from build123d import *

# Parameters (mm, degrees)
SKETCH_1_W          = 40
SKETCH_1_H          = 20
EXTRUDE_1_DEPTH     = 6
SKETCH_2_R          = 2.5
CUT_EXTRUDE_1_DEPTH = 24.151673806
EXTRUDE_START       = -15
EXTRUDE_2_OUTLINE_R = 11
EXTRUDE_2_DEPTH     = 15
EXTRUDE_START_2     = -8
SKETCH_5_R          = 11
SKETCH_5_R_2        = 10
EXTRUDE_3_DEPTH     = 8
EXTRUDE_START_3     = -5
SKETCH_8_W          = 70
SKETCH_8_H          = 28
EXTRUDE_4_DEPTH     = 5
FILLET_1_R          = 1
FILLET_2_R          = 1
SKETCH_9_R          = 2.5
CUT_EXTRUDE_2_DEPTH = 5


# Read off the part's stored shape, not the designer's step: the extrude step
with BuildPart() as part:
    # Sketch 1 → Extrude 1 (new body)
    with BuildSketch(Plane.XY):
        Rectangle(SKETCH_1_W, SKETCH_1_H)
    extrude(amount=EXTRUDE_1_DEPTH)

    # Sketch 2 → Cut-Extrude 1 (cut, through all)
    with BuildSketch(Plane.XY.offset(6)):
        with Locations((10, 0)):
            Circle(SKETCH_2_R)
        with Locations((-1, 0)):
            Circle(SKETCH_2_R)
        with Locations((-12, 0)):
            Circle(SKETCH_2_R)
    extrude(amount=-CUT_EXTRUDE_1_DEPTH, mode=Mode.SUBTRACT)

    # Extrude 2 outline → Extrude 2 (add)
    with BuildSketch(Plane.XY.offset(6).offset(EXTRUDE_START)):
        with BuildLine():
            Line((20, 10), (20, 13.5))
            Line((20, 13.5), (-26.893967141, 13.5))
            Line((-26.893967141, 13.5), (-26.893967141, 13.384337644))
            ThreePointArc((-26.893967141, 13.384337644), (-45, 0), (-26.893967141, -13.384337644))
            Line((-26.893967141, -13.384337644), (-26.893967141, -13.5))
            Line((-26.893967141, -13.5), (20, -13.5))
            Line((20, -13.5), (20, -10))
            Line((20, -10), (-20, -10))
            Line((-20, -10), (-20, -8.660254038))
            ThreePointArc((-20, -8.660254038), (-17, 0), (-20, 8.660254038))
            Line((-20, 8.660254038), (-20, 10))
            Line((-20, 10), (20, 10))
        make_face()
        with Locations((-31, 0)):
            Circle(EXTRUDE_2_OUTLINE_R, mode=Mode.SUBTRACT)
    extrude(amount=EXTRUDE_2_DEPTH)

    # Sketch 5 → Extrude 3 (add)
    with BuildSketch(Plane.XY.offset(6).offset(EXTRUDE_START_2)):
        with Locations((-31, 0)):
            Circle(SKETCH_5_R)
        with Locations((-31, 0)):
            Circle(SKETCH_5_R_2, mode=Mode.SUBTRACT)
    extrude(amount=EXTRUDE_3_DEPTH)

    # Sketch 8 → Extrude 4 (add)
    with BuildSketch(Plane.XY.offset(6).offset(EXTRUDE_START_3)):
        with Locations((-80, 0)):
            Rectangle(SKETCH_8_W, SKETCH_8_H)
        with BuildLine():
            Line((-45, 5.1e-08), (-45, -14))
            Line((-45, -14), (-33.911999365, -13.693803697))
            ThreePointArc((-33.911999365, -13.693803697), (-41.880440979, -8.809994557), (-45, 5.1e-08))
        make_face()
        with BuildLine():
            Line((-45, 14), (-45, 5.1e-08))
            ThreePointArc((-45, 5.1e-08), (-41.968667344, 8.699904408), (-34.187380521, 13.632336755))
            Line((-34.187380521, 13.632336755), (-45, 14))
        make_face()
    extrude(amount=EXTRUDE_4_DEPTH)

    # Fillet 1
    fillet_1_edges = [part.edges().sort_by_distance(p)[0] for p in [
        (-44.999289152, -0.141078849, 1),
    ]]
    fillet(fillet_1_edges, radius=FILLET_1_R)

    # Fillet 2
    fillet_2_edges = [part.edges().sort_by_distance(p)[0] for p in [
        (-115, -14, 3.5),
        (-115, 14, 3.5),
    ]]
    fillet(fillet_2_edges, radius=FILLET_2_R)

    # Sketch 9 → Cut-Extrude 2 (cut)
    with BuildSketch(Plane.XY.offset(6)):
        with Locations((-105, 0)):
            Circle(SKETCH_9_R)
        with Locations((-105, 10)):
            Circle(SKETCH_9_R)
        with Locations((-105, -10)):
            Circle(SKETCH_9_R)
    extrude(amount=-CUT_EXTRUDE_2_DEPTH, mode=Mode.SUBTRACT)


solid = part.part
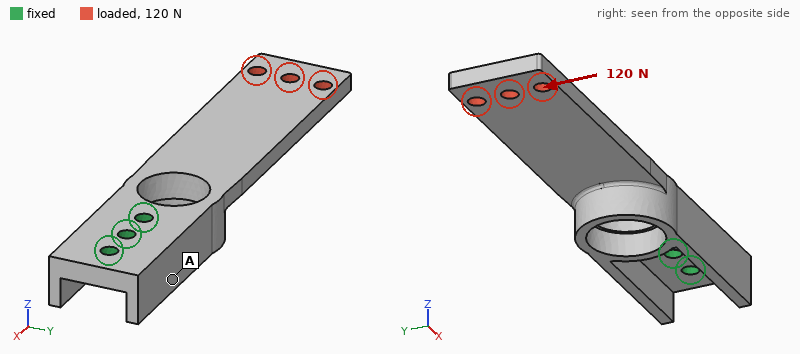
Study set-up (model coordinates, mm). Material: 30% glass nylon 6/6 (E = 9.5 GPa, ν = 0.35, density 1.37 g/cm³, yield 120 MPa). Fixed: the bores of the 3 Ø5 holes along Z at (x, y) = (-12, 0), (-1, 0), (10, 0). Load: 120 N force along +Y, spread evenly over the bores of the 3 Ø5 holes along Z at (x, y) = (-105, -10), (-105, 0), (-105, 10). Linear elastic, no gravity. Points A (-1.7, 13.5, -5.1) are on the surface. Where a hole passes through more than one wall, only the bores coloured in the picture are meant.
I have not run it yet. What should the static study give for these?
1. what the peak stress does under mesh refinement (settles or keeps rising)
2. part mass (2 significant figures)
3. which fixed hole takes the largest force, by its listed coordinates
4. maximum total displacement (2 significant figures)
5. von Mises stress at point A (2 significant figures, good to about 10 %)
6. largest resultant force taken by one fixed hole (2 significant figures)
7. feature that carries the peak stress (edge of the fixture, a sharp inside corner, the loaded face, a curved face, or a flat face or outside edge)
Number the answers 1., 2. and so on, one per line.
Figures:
1. keeps rising
2. 31 g
3. (-12, 0)
4. 0.58 mm
5. 3.2 MPa
6. 550 N
7. edge of the fixture
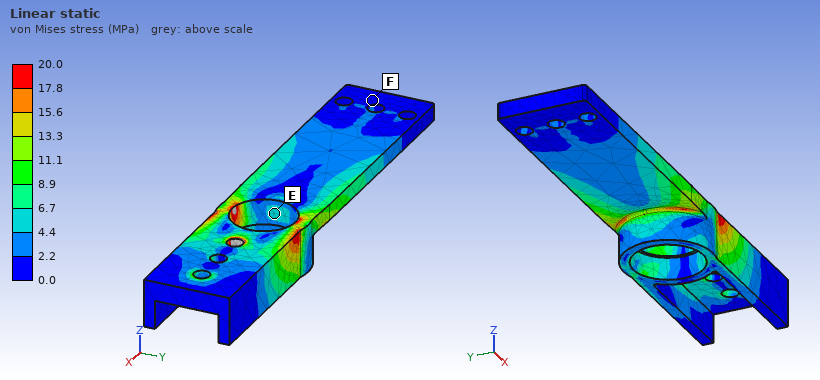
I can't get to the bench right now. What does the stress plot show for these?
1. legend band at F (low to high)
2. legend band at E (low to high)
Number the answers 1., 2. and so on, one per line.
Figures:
1. 0.0 to 2.2 MPa
2. 4.4 to 6.7 MPa
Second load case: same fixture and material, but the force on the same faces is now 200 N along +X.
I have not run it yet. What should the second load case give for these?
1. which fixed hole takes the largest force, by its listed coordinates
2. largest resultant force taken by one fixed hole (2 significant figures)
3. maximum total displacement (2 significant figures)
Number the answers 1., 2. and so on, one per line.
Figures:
1. (-12, 0)
2. 98 N
3. 0.12 mm
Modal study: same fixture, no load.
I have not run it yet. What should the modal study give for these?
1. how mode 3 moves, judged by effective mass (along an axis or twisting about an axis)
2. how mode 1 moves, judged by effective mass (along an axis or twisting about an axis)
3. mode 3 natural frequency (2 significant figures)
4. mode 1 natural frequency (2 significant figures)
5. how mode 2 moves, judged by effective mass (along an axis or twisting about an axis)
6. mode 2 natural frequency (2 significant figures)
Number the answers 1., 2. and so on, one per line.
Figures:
1. twisting about X
2. along Z
3. 1600 Hz
4. 320 Hz
5. along Y
6. 940 Hz
